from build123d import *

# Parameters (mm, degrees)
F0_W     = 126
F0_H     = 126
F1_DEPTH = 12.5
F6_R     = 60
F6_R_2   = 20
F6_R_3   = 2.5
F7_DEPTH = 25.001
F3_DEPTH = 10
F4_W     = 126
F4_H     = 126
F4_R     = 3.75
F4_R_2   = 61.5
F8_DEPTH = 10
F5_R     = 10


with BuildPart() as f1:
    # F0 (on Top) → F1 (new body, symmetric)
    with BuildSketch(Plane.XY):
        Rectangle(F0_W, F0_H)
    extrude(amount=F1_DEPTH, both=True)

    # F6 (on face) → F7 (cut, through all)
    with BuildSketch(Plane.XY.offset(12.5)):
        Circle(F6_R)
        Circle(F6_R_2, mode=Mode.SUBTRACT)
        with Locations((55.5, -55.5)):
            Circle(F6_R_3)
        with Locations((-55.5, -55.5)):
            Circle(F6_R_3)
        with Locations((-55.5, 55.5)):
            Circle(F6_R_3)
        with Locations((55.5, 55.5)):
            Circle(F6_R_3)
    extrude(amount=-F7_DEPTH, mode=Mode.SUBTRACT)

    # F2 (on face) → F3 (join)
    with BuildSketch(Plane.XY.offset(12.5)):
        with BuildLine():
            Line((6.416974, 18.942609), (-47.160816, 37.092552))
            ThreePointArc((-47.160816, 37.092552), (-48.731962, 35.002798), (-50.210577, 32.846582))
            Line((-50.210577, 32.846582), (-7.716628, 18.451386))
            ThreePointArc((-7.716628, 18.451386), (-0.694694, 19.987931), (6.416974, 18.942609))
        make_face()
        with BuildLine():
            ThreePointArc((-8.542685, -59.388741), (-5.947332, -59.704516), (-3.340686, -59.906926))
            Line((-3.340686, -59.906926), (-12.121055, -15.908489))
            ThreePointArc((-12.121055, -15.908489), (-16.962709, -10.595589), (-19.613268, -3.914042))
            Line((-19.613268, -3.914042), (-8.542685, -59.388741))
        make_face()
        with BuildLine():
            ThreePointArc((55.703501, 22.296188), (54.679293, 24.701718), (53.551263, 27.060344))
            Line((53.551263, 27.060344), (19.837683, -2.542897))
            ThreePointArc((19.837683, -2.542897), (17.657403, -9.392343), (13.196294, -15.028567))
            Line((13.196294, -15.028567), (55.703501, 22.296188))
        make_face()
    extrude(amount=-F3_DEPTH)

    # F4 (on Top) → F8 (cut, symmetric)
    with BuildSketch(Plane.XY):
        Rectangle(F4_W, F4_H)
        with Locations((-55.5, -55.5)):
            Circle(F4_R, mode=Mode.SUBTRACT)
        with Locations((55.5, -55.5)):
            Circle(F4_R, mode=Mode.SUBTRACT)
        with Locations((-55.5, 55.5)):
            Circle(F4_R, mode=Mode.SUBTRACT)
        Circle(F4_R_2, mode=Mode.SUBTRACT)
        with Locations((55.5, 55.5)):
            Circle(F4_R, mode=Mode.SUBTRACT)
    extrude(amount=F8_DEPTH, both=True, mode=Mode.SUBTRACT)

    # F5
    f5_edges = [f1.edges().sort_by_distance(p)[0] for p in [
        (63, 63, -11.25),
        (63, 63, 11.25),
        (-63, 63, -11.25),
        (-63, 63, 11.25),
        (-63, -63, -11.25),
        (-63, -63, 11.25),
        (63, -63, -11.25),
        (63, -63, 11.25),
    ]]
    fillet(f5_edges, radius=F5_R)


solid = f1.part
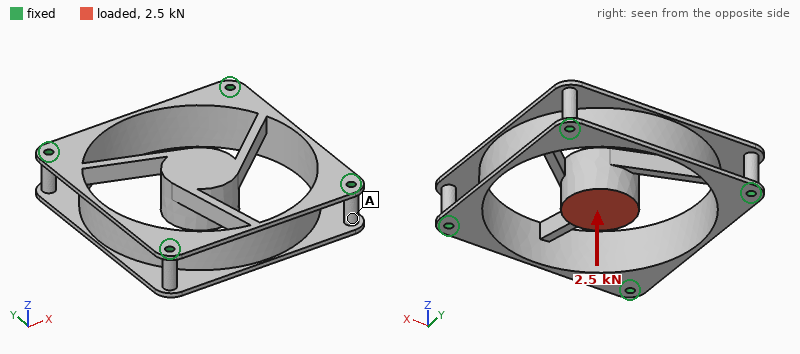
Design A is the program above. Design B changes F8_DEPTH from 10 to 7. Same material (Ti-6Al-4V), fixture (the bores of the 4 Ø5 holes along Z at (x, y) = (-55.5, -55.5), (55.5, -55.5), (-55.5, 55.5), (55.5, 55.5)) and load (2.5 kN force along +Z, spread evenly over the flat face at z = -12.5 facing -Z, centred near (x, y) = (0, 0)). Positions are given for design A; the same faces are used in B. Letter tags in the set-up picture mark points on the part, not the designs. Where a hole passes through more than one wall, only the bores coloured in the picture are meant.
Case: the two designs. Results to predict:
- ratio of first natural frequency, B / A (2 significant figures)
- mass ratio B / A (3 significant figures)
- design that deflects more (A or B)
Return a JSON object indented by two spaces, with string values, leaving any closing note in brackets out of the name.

{
  "ratio of first natural frequency, B / A": "1.2",
  "mass ratio B / A": "1.30",
  "design that deflects more": "A"
}
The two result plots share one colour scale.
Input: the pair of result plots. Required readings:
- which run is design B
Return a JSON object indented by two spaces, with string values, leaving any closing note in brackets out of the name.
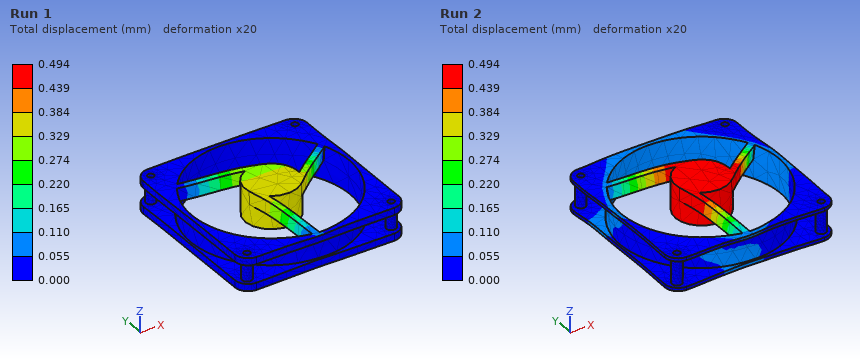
{
  "which run is design B": "Run 1"
}
